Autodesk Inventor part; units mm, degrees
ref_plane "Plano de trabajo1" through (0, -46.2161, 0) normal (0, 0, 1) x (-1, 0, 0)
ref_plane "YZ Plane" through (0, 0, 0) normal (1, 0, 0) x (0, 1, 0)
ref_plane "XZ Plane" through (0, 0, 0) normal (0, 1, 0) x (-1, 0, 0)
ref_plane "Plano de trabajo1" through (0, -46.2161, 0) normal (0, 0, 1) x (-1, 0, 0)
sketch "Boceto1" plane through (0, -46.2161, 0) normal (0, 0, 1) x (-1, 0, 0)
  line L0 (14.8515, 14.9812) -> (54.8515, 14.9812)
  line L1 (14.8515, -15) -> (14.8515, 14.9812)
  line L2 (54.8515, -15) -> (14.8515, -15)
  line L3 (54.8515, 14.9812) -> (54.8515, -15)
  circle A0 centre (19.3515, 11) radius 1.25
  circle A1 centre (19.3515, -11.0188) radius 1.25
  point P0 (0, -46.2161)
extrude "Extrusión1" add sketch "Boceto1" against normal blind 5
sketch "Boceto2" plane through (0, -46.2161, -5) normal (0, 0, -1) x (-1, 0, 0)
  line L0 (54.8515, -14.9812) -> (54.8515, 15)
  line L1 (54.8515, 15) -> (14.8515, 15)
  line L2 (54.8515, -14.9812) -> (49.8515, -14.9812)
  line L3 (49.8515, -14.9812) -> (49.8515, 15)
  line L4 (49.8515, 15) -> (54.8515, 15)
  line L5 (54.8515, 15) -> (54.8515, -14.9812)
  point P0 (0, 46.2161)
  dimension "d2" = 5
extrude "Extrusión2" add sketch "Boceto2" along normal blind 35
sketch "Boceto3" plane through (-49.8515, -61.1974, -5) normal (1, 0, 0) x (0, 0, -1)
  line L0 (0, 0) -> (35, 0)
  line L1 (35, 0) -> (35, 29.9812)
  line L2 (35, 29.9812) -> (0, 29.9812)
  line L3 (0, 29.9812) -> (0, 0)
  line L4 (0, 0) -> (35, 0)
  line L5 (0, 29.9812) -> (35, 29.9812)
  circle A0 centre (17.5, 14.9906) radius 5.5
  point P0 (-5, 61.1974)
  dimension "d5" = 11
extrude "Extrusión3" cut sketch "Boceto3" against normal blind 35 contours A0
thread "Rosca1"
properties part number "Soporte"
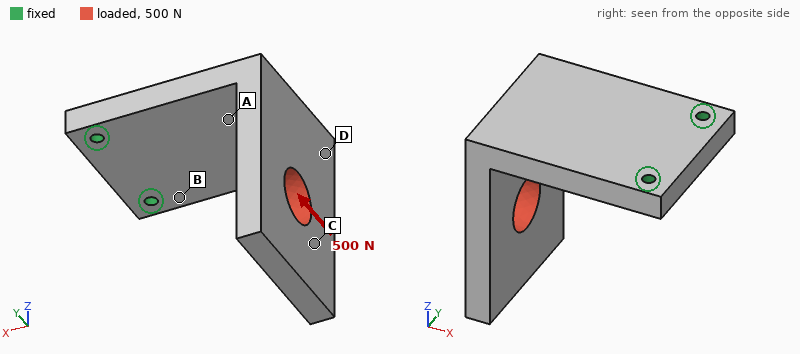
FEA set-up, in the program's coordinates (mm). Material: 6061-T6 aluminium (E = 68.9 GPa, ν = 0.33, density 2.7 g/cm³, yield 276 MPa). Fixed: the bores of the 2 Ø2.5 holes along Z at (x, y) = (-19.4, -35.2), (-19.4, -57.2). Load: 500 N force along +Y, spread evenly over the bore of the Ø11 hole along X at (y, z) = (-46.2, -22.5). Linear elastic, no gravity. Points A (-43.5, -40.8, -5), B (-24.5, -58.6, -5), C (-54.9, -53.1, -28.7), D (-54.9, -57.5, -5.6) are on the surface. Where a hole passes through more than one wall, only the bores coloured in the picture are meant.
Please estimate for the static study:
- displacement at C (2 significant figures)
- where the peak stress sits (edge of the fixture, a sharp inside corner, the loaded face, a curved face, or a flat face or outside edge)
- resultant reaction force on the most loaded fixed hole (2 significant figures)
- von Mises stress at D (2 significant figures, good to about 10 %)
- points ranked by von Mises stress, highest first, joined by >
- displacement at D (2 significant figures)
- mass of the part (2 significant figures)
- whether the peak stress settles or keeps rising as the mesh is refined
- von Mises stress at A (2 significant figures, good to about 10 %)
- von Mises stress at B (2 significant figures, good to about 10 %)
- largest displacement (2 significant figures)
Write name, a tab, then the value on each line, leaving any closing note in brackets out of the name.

displacement at C	0.22 mm
where the peak stress sits	edge of the fixture
resultant reaction force on the most loaded fixed hole	870 N
von Mises stress at D	26 MPa
points ranked by von Mises stress, highest first, joined by >	A > B > D > C
displacement at D	0.096 mm
mass of the part	29 g
whether the peak stress settles or keeps rising as the mesh is refined	keeps rising
von Mises stress at A	67 MPa
von Mises stress at B	47 MPa
largest displacement	0.33 mm
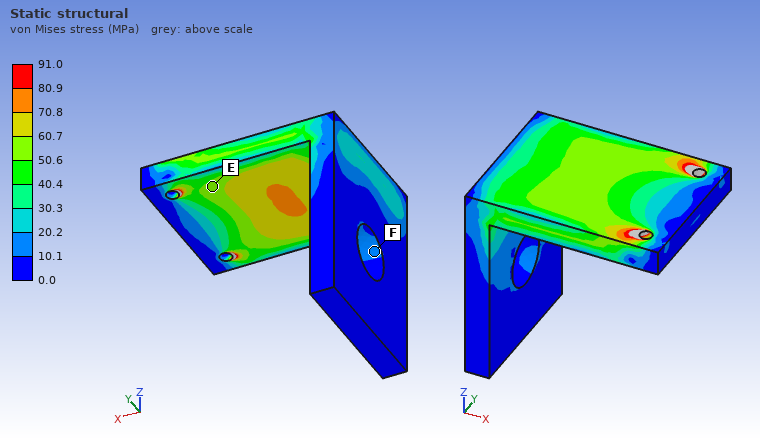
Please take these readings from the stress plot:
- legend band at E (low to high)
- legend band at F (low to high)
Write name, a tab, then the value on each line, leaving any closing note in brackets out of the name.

legend band at E	50.6 to 60.7 MPa
legend band at F	10.1 to 20.2 MPa
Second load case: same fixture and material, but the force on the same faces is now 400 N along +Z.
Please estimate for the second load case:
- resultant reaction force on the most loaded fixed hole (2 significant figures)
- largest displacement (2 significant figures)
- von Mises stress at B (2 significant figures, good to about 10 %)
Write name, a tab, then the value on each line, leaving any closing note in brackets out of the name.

resultant reaction force on the most loaded fixed hole	200 N
largest displacement	0.51 mm
von Mises stress at B	110 MPa
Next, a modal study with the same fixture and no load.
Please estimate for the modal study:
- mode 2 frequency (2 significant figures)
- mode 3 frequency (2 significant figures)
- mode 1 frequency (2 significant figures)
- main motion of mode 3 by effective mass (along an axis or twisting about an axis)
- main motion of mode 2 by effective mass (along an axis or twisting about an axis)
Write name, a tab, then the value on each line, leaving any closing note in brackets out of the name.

mode 2 frequency	2000 Hz
mode 3 frequency	3000 Hz
mode 1 frequency	1100 Hz
main motion of mode 3 by effective mass	along Z
main motion of mode 2 by effective mass	along Y
